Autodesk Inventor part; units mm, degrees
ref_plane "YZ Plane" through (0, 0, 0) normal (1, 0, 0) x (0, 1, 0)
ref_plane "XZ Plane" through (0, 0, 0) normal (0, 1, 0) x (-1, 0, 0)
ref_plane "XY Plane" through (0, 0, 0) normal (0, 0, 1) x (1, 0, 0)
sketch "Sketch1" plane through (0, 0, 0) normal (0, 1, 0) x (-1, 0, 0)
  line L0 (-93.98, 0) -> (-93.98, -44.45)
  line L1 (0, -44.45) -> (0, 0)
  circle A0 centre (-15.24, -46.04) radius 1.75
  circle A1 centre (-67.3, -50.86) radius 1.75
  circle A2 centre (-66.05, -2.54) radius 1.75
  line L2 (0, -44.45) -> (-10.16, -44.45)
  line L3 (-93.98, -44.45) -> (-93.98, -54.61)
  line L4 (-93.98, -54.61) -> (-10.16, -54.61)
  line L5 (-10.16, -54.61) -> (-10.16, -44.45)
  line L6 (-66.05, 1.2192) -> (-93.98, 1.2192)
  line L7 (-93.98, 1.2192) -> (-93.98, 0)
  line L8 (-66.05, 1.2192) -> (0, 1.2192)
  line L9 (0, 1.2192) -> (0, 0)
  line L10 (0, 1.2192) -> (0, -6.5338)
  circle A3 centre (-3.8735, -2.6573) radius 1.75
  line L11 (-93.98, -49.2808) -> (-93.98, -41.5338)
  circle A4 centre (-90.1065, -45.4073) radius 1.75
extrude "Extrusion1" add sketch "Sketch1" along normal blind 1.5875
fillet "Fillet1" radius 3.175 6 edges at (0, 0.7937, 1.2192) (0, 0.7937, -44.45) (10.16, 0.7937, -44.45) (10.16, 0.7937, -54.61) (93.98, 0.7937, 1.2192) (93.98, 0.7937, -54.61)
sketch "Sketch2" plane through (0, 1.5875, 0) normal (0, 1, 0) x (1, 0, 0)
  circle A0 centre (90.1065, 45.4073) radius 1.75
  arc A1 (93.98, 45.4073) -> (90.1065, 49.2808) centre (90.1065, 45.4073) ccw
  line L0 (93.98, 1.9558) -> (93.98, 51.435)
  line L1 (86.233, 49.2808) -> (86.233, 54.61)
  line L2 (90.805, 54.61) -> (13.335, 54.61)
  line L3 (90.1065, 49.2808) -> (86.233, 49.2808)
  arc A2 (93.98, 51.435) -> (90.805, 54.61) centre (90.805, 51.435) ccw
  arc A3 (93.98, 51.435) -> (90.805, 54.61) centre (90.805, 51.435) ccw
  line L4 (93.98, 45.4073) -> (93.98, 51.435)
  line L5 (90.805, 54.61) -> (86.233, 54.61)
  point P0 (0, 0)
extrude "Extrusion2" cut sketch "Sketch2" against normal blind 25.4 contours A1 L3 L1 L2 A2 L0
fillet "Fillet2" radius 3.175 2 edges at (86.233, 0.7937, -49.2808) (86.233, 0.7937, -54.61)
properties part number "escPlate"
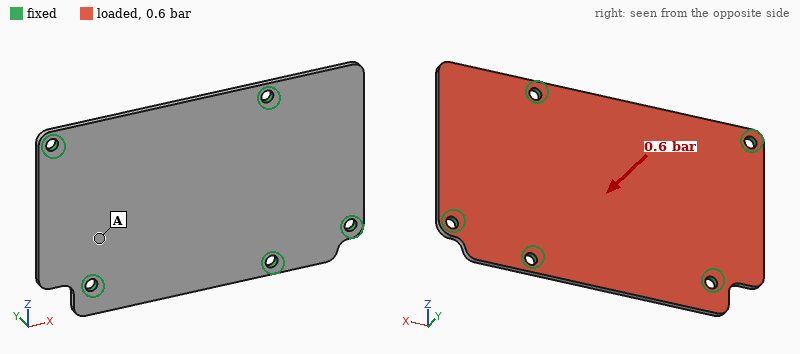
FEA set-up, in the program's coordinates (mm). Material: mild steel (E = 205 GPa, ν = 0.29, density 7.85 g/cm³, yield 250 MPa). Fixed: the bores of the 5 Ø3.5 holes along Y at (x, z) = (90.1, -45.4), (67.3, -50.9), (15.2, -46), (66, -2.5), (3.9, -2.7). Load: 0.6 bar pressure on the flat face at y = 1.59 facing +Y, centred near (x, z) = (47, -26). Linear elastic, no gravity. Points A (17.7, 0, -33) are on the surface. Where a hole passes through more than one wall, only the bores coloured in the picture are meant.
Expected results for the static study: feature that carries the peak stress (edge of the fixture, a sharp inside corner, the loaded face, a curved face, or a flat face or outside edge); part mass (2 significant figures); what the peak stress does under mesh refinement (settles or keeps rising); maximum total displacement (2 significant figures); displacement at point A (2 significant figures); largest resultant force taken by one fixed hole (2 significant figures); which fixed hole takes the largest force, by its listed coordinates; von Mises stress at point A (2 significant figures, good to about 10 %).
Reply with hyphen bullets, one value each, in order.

- edge of the fixture
- 63 g
- keeps rising
- 38 µm
- 14 µm
- 90 N
- (66, -2.5)
- 13 MPa
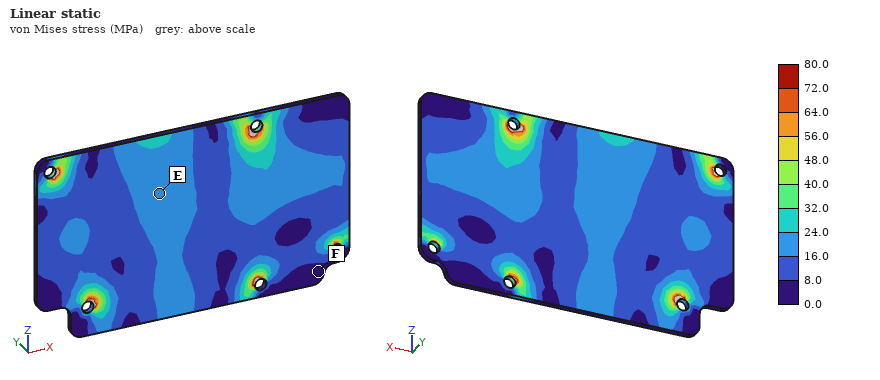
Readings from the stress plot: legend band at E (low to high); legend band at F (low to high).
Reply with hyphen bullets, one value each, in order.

- 16.0 to 24.0 MPa
- 0.0 to 8.0 MPa
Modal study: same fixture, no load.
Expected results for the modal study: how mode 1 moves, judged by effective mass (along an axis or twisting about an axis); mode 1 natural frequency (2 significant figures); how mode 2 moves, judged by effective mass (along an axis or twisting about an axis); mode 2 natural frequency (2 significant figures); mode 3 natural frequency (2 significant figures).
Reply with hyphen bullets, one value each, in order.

- along Y
- 2100 Hz
- along Y
- 2300 Hz
- 3200 Hz
